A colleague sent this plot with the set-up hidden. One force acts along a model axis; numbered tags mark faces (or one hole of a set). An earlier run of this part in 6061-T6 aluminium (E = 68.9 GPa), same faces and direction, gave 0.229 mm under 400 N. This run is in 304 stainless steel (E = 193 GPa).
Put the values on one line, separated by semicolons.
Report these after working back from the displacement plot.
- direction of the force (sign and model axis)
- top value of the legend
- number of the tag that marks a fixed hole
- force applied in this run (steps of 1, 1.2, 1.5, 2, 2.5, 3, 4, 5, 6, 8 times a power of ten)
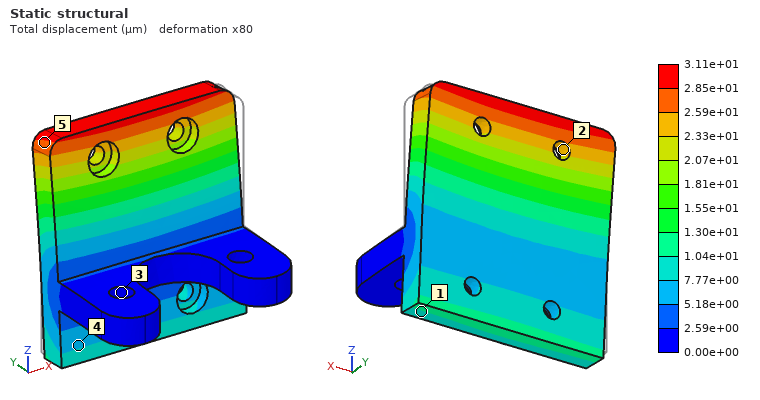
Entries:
+Y; 3.11e+01 µm; 3; 150 N
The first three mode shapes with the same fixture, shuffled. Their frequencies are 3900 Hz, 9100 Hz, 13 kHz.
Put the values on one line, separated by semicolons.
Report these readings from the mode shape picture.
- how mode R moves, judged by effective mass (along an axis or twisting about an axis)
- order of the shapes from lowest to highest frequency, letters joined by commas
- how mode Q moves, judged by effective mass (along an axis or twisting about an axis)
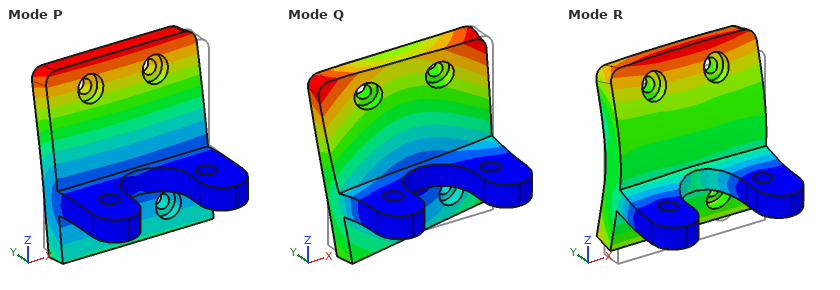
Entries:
along Z; P, Q, R; along X
